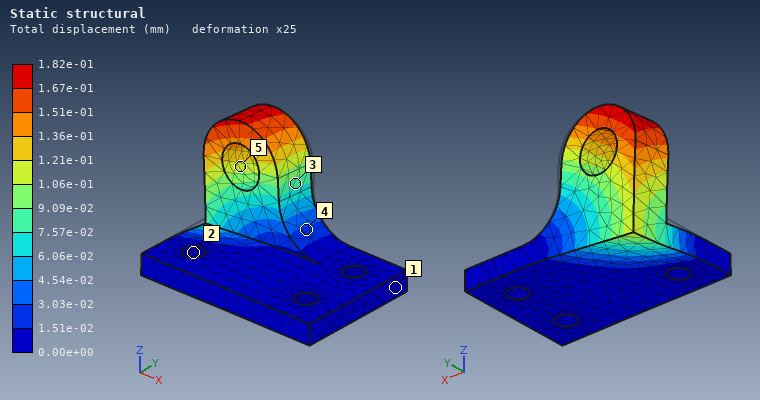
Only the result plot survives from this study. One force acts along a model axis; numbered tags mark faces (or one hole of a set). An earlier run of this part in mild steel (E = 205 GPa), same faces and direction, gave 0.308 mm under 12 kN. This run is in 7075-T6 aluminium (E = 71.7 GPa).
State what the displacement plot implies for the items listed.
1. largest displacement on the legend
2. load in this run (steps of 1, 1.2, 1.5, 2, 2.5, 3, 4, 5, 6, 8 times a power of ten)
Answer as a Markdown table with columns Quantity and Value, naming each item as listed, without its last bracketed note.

| Quantity | Value |
|---|---|
| largest displacement on the legend | 1.82e-01 mm |
| load in this run | 2.5 kN |
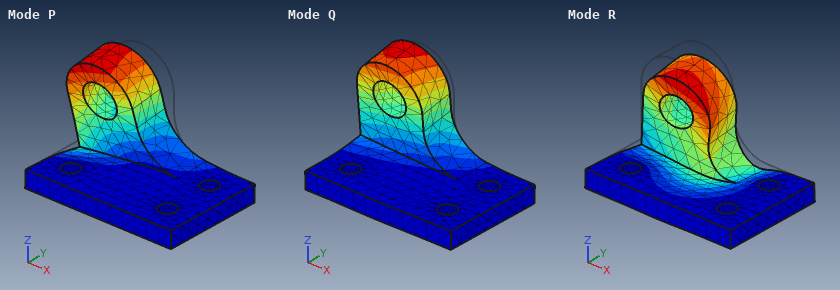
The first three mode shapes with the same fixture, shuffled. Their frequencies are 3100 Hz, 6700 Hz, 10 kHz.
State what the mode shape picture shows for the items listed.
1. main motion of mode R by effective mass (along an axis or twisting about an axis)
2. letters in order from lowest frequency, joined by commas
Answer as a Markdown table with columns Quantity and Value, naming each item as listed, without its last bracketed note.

| Quantity | Value |
|---|---|
| main motion of mode R by effective mass | along Z |
| letters in order from lowest frequency, joined by commas | Q, P, R |
